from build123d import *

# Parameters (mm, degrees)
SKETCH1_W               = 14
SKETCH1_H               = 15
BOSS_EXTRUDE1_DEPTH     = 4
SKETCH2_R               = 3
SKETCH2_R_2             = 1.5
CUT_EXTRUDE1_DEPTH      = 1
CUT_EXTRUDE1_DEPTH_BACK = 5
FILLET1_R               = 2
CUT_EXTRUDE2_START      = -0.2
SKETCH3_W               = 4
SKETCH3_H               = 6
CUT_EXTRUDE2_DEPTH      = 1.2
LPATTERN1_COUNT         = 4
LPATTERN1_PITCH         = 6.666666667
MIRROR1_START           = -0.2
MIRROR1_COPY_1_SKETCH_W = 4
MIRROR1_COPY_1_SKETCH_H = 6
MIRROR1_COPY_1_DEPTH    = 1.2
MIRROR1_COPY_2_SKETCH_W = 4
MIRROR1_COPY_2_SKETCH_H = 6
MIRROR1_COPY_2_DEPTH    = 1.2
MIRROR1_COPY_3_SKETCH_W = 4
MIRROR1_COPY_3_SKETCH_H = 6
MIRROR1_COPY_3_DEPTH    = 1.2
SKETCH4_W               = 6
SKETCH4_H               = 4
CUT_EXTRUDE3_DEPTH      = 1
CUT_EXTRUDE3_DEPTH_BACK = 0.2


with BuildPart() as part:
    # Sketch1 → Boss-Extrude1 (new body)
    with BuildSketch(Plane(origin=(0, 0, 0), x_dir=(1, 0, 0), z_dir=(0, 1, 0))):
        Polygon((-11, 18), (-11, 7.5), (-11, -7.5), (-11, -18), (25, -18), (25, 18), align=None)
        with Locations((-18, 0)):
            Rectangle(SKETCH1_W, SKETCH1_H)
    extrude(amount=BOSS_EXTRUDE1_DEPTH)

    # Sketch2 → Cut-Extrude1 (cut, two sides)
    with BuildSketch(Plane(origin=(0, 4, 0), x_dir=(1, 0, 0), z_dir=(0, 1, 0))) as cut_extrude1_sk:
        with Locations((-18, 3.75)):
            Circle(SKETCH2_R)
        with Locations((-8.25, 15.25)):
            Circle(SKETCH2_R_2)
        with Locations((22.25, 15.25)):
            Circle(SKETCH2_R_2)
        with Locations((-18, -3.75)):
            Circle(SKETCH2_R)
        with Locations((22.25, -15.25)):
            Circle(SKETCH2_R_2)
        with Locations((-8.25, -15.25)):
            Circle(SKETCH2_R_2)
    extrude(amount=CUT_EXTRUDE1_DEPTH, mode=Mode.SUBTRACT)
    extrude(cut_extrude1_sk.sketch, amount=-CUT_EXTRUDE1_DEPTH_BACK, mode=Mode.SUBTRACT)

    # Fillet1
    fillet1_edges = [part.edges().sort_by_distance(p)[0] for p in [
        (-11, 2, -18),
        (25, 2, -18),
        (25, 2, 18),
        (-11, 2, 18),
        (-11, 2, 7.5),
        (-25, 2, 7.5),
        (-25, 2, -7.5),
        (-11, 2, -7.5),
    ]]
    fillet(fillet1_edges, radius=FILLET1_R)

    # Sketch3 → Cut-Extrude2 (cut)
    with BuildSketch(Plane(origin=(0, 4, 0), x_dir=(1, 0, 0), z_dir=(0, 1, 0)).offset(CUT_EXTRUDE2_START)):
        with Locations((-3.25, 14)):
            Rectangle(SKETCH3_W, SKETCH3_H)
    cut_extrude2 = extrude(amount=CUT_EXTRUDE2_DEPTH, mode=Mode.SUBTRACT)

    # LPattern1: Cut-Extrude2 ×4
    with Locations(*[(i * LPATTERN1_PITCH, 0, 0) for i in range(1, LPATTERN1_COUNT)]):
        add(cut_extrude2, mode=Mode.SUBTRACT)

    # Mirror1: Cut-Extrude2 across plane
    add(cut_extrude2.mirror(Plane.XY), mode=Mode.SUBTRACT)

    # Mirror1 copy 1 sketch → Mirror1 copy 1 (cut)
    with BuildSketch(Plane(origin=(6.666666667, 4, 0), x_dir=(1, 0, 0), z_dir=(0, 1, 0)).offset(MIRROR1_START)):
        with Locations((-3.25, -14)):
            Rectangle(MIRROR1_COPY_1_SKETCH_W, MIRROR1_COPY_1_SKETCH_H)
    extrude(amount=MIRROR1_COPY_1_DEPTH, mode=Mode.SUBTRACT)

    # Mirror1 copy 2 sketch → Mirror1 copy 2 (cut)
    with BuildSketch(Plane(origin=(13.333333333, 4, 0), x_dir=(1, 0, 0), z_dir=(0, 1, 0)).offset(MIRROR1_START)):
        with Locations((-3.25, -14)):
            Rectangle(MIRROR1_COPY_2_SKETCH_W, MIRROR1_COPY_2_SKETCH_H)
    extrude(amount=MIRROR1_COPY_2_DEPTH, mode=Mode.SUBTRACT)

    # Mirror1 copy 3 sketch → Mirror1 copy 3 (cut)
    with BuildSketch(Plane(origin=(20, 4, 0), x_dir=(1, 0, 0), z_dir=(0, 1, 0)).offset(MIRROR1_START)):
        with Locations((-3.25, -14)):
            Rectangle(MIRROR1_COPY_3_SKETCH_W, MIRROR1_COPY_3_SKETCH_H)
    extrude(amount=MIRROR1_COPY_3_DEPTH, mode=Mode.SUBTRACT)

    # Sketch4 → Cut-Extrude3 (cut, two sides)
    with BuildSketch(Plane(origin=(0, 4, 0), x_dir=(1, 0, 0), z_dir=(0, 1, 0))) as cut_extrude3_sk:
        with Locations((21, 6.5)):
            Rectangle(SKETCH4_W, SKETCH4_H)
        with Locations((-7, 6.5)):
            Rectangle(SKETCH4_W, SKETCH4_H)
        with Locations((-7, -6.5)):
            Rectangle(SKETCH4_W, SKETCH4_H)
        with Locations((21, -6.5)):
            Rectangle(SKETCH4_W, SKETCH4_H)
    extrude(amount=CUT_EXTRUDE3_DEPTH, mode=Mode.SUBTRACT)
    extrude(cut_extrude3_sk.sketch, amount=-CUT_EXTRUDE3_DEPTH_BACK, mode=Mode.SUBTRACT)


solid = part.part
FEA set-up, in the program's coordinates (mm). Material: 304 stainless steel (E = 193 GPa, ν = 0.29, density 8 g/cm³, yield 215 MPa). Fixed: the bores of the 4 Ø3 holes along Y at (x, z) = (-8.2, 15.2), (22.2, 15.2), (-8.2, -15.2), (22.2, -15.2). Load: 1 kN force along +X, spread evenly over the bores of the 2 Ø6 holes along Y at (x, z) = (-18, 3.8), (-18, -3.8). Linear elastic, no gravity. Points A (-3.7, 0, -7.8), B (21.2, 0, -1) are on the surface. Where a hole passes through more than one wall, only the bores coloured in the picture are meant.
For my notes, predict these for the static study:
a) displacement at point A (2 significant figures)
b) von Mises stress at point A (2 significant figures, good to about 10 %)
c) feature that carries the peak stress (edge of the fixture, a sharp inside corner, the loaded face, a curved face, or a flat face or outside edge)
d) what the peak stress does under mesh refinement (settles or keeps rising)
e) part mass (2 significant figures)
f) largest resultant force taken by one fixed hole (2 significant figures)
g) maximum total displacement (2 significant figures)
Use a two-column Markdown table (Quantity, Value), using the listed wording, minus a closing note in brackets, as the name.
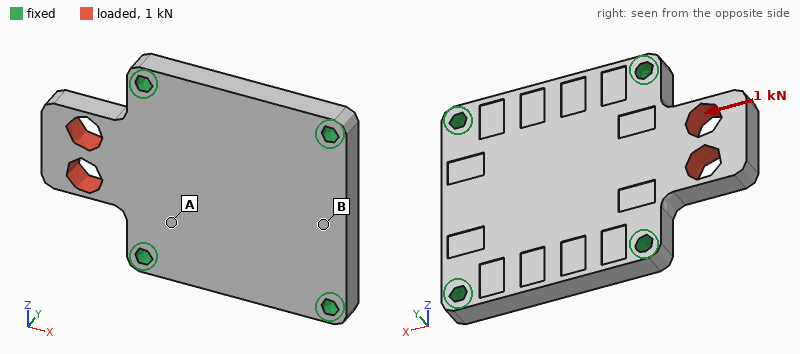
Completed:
| Quantity | Value |
|---|---|
| displacement at point A | 0.74 µm |
| von Mises stress at point A | 11 MPa |
| feature that carries the peak stress | a sharp inside corner |
| what the peak stress does under mesh refinement | keeps rising |
| part mass | 45 g |
| largest resultant force taken by one fixed hole | 300 N |
| maximum total displacement | 3.0 µm |
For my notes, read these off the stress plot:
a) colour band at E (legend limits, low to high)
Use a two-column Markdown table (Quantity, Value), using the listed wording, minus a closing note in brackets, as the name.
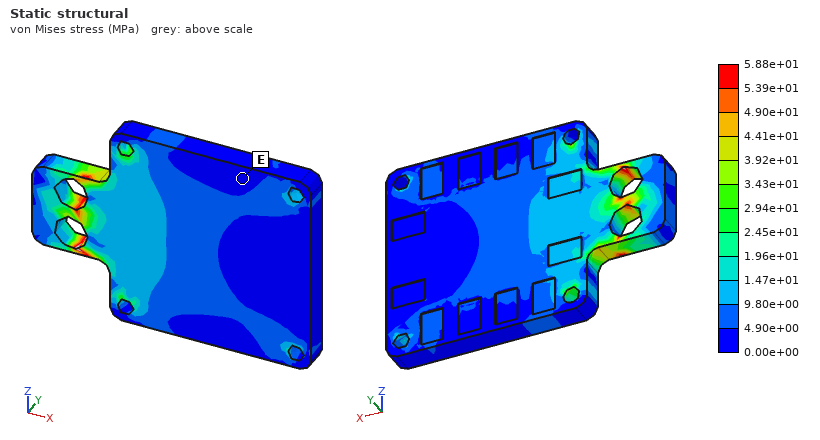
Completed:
| Quantity | Value |
|---|---|
| colour band at E | 0.00e+00 to 4.90e+00 MPa |
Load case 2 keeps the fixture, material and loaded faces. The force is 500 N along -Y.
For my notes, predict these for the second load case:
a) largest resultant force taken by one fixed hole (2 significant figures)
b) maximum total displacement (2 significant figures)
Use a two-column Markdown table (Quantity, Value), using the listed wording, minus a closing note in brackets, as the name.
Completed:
| Quantity | Value |
|---|---|
| largest resultant force taken by one fixed hole | 310 N |
| maximum total displacement | 59 µm |
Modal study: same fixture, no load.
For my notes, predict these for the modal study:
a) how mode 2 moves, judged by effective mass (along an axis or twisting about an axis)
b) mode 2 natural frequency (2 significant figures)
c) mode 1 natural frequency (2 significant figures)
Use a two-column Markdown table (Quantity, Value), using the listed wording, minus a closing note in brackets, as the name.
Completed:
| Quantity | Value |
|---|---|
| how mode 2 moves, judged by effective mass | along Y |
| mode 2 natural frequency | 14 kHz |
| mode 1 natural frequency | 7400 Hz |
